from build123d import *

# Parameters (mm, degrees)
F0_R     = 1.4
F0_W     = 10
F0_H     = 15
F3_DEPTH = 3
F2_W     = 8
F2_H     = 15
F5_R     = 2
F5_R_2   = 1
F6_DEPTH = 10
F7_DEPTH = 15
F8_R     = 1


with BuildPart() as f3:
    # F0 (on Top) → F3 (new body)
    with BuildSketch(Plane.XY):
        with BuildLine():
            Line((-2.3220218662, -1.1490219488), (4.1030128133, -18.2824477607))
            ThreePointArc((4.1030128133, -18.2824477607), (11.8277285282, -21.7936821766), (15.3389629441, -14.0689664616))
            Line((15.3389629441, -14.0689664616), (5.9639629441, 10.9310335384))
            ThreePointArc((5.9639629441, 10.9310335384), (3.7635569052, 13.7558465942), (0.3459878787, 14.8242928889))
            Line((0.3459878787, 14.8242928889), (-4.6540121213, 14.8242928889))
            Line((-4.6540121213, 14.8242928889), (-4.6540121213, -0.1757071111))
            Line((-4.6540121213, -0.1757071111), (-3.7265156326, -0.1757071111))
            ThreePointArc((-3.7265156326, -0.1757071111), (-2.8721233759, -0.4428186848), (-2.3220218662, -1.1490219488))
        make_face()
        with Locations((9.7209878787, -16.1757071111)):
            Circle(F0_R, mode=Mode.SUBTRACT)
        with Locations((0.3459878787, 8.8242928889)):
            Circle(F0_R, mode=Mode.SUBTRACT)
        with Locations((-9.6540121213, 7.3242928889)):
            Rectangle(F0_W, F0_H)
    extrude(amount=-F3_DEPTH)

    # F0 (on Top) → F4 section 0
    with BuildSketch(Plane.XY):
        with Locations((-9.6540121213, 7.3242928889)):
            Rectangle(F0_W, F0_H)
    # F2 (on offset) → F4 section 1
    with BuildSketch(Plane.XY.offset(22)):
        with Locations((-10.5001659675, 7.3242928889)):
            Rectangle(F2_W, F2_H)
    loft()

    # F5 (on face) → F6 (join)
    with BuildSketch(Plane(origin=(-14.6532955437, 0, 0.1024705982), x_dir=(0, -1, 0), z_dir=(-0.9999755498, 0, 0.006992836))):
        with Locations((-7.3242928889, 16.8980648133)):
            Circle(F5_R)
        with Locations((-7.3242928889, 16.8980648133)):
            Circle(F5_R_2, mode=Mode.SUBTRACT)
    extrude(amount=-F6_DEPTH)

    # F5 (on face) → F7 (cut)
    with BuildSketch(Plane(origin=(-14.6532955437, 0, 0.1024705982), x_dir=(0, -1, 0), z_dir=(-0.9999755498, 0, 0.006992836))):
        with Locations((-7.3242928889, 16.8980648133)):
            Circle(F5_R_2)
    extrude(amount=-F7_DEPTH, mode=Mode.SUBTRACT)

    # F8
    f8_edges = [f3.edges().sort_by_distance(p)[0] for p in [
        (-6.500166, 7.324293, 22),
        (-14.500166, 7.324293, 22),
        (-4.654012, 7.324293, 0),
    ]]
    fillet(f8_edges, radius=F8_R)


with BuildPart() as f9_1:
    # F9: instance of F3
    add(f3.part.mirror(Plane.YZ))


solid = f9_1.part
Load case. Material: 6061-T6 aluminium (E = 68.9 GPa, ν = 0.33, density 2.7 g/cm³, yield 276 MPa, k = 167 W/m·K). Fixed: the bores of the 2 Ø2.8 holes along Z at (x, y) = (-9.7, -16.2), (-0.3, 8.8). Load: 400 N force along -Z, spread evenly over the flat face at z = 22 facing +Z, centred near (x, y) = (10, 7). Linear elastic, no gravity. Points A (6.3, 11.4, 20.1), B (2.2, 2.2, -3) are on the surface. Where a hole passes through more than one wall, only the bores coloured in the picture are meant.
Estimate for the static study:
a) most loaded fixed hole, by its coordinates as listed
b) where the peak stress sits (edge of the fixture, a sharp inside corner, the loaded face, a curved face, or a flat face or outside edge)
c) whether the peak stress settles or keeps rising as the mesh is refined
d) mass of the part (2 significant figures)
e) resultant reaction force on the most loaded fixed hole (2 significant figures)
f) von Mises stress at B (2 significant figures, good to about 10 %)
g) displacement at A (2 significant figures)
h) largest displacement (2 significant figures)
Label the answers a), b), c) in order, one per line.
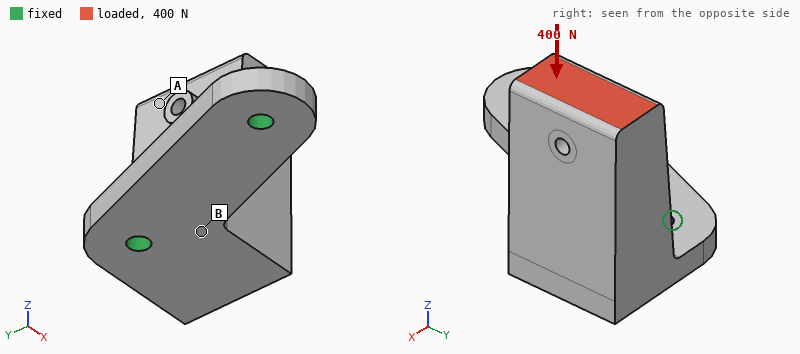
a) (-0.3, 8.8)
b) edge of the fixture
c) keeps rising
d) 13 g
e) 420 N
f) 92 MPa
g) 0.18 mm
h) 0.22 mm
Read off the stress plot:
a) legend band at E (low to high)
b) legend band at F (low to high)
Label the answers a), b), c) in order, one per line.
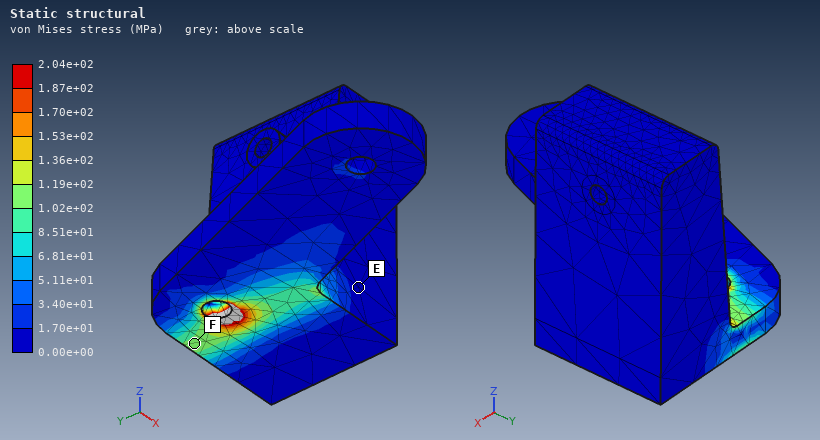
a) 0.00e+00 to 1.70e+01 MPa
b) 1.02e+02 to 1.19e+02 MPa
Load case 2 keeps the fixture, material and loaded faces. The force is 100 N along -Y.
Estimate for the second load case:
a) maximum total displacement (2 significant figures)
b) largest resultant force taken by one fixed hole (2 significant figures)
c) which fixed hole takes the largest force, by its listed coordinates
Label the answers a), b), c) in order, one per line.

a) 77 µm
b) 99 N
c) (-0.3, 8.8)
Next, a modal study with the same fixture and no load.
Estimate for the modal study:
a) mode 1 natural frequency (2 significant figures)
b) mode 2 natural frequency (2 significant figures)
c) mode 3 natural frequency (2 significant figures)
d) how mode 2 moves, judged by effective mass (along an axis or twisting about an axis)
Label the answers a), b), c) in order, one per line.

a) 2100 Hz
b) 3500 Hz
c) 13 kHz
d) along Y
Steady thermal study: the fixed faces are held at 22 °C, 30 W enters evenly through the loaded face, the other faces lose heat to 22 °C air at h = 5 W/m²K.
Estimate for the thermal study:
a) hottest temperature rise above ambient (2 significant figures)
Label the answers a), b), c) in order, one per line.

a) 63 K
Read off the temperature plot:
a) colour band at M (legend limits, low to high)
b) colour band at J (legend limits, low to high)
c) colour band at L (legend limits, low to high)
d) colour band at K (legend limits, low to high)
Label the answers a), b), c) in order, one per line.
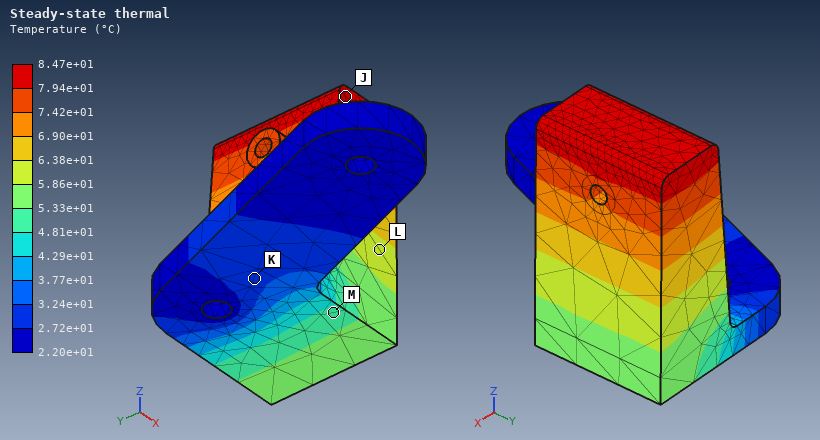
a) 4.81e+01 to 5.33e+01 °C
b) 7.94e+01 to 8.47e+01 °C
c) 5.86e+01 to 6.38e+01 °C
d) 2.72e+01 to 3.24e+01 °C
